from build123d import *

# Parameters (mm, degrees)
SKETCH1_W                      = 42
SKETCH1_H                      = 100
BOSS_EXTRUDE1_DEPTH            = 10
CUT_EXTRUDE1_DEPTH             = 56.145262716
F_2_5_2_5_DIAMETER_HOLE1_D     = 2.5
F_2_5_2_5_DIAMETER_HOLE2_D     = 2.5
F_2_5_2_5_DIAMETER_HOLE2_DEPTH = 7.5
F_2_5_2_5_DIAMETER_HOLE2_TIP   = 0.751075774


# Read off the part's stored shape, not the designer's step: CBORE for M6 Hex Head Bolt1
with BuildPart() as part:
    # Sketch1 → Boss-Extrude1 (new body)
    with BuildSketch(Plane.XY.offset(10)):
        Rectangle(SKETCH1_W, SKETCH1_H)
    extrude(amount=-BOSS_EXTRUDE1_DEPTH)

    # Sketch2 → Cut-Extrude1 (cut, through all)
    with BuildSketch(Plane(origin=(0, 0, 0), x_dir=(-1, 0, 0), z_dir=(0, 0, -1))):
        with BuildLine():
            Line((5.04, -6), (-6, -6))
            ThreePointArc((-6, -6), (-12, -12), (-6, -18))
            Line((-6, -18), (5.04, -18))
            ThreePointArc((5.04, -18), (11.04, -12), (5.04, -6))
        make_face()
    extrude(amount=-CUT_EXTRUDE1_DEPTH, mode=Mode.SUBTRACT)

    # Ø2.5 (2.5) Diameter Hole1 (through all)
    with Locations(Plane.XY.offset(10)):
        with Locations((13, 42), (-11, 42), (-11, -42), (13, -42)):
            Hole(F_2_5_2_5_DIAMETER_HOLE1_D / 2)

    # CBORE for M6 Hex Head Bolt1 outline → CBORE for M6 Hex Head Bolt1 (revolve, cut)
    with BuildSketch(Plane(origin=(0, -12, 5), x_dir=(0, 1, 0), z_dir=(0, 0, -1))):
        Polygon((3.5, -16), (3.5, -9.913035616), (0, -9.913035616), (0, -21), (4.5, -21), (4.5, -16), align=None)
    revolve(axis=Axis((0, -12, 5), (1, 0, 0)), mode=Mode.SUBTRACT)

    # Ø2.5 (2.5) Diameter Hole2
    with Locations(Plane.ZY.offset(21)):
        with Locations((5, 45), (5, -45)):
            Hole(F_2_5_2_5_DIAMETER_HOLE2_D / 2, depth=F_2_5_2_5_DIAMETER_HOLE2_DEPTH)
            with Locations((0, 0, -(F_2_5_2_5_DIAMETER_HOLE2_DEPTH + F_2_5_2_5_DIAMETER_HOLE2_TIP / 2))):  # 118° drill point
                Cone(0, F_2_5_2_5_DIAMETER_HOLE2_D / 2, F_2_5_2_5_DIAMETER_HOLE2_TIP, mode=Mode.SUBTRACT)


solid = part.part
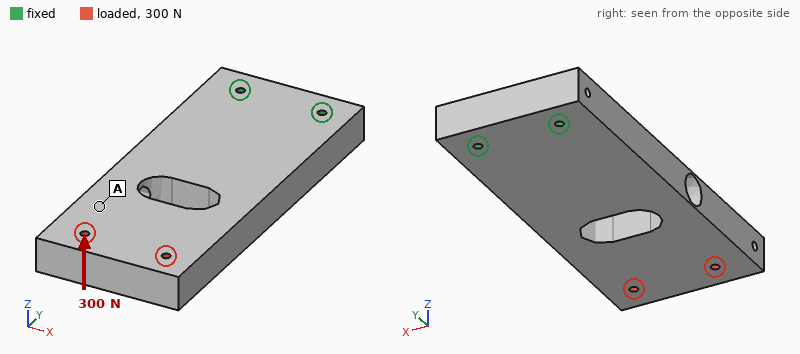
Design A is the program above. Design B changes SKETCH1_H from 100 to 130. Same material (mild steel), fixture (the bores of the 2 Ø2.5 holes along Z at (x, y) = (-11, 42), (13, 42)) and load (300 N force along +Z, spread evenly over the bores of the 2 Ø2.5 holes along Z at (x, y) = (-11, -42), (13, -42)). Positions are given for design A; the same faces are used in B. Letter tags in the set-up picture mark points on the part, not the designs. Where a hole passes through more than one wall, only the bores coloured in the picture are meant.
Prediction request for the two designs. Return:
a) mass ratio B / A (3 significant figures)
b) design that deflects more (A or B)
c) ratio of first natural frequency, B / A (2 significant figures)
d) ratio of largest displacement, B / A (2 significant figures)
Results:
1.33
B
0.72
1.2
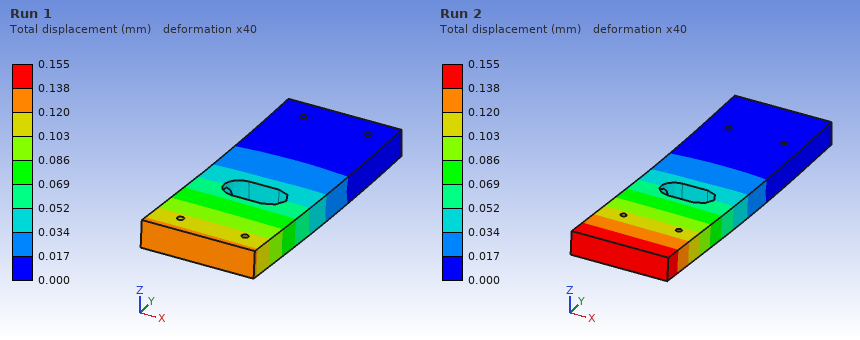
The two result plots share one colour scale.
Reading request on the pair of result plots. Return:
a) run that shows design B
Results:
Run 2
